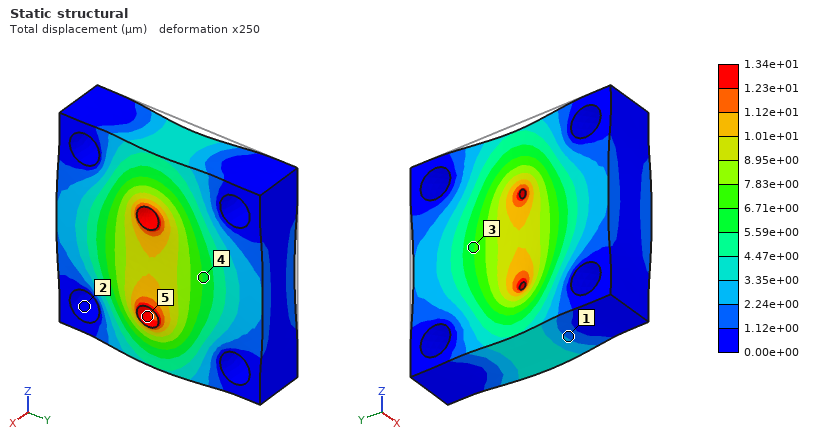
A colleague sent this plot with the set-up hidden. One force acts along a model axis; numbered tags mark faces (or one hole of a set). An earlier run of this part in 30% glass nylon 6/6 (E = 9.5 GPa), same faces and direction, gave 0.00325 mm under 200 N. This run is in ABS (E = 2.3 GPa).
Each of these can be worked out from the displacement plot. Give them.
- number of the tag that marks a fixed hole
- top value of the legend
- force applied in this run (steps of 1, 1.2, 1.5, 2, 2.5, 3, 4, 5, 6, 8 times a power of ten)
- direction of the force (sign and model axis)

2
1.34e+01 µm
200 N
+X
